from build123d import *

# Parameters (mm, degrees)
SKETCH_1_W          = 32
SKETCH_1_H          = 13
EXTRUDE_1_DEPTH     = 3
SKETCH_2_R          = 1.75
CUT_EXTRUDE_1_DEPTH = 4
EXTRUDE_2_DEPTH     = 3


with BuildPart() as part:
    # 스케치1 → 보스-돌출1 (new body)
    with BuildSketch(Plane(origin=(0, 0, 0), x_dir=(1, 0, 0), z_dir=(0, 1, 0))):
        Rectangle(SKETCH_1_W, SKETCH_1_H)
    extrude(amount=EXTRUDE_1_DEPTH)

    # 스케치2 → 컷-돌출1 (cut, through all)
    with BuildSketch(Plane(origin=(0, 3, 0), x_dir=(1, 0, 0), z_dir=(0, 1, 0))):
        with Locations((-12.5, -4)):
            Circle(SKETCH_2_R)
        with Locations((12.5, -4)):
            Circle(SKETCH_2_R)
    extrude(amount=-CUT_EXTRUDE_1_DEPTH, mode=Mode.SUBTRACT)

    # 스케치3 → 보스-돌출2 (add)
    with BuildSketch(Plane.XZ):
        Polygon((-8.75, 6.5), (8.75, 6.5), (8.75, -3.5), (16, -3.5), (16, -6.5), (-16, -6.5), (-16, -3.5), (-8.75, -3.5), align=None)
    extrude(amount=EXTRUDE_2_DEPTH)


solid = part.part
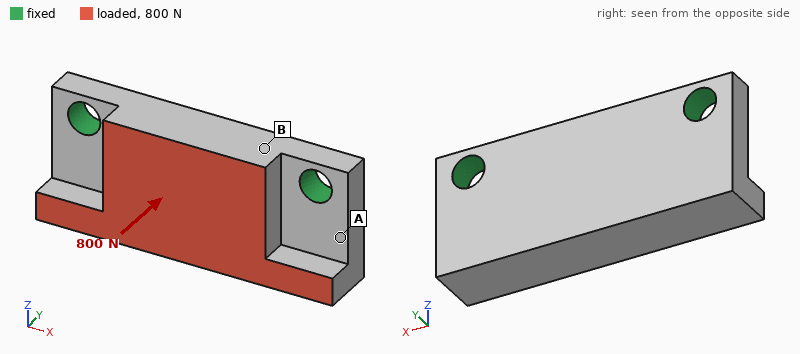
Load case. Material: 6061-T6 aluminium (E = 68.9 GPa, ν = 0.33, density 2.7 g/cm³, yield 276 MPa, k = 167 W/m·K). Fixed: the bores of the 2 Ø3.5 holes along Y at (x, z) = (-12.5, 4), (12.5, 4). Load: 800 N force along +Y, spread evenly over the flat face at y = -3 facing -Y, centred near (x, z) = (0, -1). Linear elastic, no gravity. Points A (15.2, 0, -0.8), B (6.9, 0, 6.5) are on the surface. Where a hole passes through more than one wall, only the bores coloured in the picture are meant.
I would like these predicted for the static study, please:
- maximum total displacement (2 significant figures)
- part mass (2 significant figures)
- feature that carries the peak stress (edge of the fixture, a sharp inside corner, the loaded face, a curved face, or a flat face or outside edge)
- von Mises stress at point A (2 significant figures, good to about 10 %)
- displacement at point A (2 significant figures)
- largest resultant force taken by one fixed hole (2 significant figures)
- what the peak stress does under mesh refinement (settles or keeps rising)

34 µm
5.4 g
edge of the fixture
39 MPa
6.2 µm
430 N
keeps rising
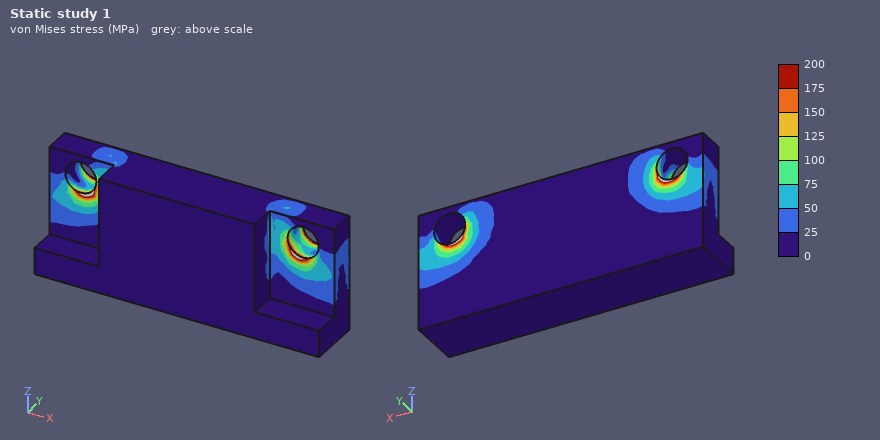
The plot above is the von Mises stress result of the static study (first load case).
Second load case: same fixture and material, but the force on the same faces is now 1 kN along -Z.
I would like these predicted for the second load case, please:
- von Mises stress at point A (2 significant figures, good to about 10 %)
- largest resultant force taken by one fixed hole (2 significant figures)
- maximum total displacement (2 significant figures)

62 MPa
540 N
46 µm
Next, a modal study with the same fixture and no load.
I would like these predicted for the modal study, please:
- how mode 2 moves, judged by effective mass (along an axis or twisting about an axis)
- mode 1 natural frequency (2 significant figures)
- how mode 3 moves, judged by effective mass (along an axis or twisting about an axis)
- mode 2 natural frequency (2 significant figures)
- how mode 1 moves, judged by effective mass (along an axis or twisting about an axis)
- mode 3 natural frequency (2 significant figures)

twisting about Z
13 kHz
along Y
29 kHz
along Y
32 kHz
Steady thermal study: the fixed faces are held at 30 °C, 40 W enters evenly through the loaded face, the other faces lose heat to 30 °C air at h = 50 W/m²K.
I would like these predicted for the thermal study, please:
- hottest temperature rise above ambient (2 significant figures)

25 K
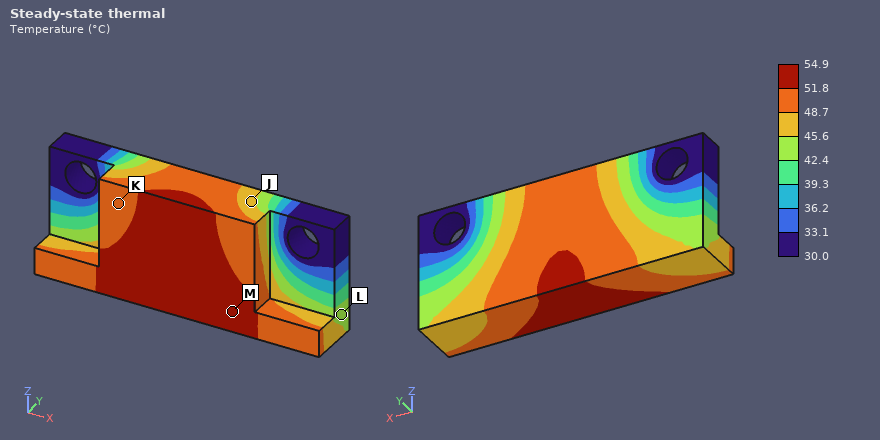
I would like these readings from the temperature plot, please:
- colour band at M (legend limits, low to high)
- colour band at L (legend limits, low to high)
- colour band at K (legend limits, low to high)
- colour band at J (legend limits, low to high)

51.8 to 54.9 °C
42.4 to 45.6 °C
48.7 to 51.8 °C
45.6 to 48.7 °C
